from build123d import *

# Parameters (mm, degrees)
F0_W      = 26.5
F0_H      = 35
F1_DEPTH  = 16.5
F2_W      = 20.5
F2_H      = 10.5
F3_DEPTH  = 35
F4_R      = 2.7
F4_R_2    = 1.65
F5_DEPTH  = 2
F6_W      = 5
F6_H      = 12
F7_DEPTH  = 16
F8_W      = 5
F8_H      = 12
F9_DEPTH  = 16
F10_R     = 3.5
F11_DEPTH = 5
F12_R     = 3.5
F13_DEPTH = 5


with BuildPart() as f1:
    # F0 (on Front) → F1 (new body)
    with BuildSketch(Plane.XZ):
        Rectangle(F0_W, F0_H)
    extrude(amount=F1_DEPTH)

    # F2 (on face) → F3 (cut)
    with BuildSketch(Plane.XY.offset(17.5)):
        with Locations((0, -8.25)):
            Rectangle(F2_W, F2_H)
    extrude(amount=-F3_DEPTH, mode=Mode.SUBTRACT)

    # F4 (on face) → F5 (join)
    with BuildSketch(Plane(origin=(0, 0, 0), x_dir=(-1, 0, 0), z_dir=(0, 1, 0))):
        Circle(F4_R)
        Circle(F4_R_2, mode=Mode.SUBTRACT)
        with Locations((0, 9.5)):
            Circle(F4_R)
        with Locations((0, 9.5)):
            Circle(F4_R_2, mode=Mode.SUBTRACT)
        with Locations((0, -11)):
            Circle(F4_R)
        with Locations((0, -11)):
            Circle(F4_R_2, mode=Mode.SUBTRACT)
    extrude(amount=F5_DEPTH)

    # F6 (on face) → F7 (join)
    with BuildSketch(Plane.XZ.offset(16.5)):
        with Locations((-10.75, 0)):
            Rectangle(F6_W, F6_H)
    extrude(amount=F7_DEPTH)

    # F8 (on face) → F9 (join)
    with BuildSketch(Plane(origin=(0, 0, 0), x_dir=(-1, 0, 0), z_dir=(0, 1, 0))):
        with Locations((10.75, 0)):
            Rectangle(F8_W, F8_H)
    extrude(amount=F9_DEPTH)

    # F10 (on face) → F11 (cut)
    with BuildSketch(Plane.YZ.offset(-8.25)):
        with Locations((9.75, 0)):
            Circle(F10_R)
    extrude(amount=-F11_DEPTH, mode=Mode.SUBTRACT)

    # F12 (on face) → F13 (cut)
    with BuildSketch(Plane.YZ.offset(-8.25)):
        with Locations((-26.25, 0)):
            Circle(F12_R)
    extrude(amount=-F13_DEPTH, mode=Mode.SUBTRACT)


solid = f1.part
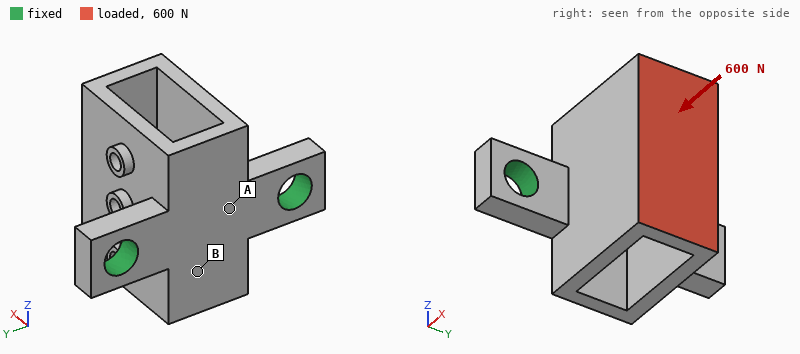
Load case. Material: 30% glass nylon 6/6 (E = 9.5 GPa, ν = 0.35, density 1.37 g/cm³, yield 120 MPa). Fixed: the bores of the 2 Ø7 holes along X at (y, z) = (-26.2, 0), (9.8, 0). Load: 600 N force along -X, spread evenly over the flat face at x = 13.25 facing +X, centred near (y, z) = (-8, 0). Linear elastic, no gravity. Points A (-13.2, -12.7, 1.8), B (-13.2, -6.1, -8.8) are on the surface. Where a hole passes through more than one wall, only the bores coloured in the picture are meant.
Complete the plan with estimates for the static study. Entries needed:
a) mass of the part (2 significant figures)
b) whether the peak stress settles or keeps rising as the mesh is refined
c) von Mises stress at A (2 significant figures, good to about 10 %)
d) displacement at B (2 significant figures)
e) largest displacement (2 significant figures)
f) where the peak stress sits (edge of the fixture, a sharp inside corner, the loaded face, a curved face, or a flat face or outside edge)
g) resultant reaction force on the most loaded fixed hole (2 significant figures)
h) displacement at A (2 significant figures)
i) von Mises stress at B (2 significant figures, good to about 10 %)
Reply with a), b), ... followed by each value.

a) 13 g
b) keeps rising
c) 11 MPa
d) 48 µm
e) 59 µm
f) edge of the fixture
g) 300 N
h) 44 µm
i) 4.8 MPa
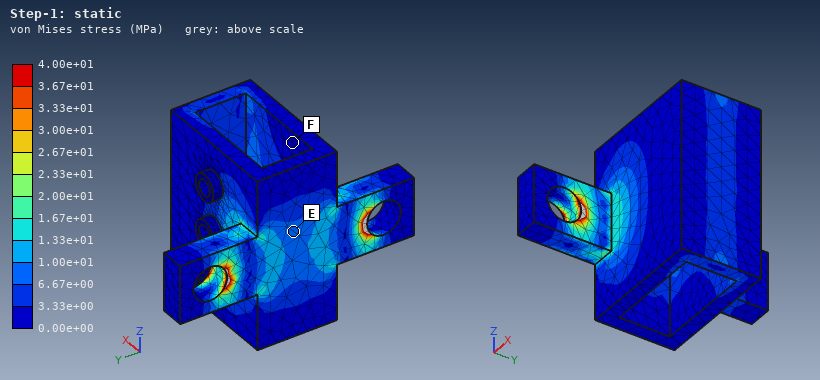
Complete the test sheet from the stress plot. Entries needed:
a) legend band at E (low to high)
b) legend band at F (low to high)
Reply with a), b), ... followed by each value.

a) 6.67e+00 to 1.00e+01 MPa
b) 0.00e+00 to 3.33e+00 MPa
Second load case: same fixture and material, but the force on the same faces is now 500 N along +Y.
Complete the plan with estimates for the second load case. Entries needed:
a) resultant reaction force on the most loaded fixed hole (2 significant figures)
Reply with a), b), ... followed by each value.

a) 550 N
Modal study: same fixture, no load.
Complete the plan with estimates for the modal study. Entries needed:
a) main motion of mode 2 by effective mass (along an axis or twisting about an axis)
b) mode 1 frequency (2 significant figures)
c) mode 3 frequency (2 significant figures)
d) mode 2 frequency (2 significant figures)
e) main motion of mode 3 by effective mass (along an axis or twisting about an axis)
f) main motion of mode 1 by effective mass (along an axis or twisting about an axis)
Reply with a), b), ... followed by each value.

a) along Y
b) 1700 Hz
c) 4400 Hz
d) 2600 Hz
e) twisting about X
f) along Z
